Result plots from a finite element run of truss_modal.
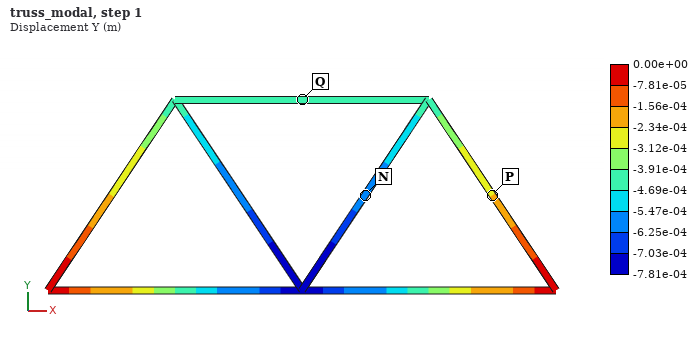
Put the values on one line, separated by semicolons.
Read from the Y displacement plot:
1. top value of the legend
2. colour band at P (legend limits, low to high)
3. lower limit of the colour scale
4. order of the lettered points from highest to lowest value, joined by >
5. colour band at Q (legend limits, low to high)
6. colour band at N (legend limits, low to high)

0.00e+00 m; -2.34e-04 to -1.56e-04 m; -7.81e-04 m; P > Q > N; -4.69e-04 to -3.91e-04 m; -6.25e-04 to -5.47e-04 m
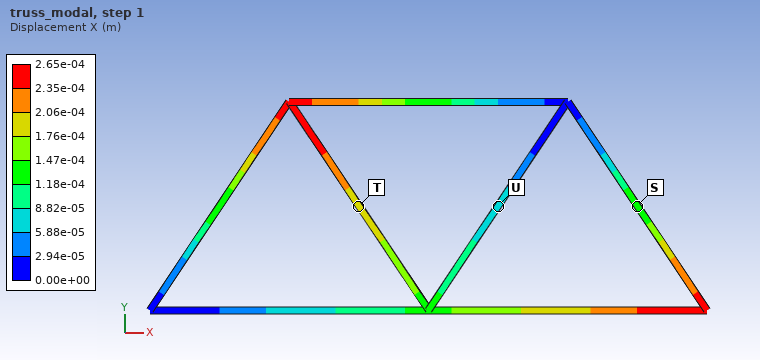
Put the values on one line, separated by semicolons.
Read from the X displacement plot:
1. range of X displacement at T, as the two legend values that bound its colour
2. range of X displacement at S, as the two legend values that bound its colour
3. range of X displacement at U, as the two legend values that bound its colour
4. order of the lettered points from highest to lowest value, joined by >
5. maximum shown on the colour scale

1.76e-04 to 2.06e-04 m; 1.18e-04 to 1.47e-04 m; 5.88e-05 to 8.82e-05 m; T > S > U; 2.65e-04 m
